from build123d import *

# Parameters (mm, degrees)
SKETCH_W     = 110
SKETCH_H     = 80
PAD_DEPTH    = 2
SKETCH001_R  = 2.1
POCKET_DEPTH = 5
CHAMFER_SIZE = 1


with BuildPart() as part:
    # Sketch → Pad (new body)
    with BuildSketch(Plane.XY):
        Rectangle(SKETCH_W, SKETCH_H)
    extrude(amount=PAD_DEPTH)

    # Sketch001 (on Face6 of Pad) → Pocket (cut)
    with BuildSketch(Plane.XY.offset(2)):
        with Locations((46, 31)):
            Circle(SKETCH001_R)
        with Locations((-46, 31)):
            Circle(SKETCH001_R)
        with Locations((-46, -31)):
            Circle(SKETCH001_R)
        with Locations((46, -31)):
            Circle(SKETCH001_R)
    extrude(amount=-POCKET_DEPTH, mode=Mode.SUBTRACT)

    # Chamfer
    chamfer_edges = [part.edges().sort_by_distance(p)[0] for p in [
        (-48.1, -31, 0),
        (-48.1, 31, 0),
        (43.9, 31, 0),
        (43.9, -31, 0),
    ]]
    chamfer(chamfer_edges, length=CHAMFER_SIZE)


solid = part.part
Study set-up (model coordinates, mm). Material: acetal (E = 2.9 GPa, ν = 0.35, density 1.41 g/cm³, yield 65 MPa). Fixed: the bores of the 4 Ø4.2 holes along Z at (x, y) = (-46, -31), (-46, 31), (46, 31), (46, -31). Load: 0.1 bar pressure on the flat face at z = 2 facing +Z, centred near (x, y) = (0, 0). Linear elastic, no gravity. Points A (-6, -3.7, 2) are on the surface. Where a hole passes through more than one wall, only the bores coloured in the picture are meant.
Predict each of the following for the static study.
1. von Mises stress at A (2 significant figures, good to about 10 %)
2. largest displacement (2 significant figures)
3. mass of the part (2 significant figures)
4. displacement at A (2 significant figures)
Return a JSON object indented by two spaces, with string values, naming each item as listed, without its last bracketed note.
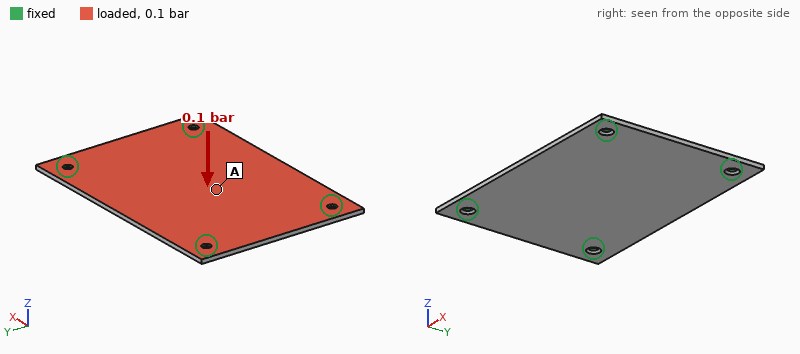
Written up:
{
  "von Mises stress at A": "5.3 MPa",
  "largest displacement": "1.5 mm",
  "mass of the part": "25 g",
  "displacement at A": "1.5 mm"
}
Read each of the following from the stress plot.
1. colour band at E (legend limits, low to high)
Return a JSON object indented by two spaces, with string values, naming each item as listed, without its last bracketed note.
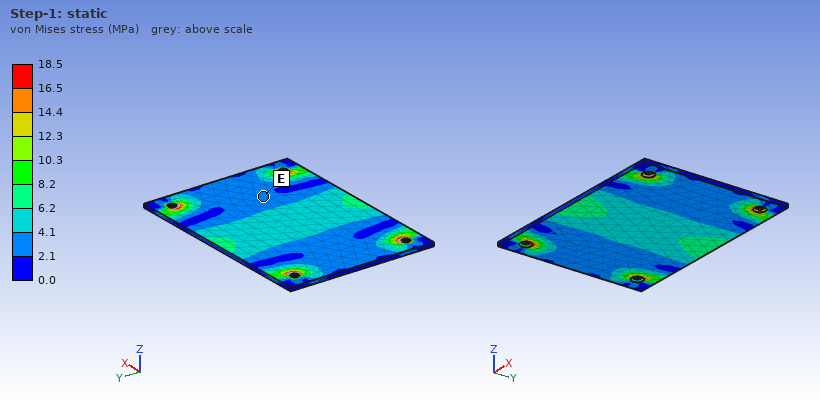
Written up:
{
  "colour band at E": "2.1 to 4.1 MPa"
}
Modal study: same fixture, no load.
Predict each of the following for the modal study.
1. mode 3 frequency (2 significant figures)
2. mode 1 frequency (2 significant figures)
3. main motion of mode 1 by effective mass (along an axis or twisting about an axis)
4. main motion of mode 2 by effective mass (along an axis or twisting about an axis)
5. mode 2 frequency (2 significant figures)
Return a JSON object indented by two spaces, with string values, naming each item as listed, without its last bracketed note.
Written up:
{
  "mode 3 frequency": "650 Hz",
  "mode 1 frequency": "280 Hz",
  "main motion of mode 1 by effective mass": "along Z",
  "main motion of mode 2 by effective mass": "twisting about X",
  "mode 2 frequency": "420 Hz"
}
